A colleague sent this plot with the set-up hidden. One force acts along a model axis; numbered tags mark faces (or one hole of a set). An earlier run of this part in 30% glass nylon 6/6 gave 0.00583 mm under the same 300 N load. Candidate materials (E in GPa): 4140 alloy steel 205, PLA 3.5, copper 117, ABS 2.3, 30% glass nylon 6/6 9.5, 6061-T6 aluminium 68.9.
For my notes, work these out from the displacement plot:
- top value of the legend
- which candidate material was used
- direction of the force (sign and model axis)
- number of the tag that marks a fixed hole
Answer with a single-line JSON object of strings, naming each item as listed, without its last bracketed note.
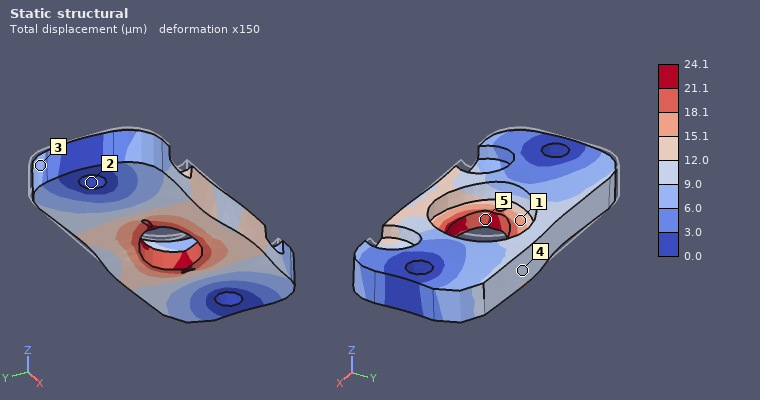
{"top value of the legend": "24.1 µm", "which candidate material was used": "ABS", "direction of the force": "+X", "number of the tag that marks a fixed hole": "2"}
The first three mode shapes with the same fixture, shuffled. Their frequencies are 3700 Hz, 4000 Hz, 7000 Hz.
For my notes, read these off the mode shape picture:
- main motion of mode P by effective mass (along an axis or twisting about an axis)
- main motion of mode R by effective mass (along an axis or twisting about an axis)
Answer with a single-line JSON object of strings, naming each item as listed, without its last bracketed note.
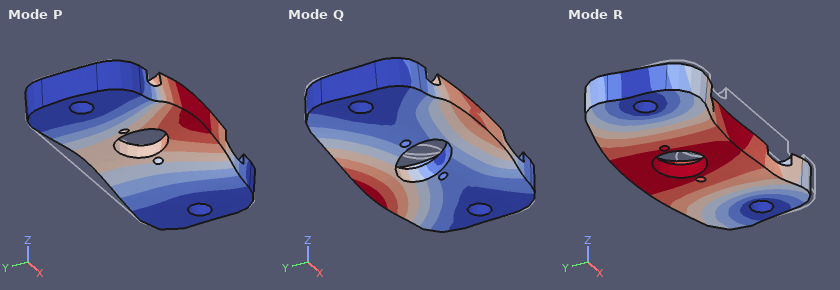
{"main motion of mode P by effective mass": "along Z", "main motion of mode R by effective mass": "along Y"}
